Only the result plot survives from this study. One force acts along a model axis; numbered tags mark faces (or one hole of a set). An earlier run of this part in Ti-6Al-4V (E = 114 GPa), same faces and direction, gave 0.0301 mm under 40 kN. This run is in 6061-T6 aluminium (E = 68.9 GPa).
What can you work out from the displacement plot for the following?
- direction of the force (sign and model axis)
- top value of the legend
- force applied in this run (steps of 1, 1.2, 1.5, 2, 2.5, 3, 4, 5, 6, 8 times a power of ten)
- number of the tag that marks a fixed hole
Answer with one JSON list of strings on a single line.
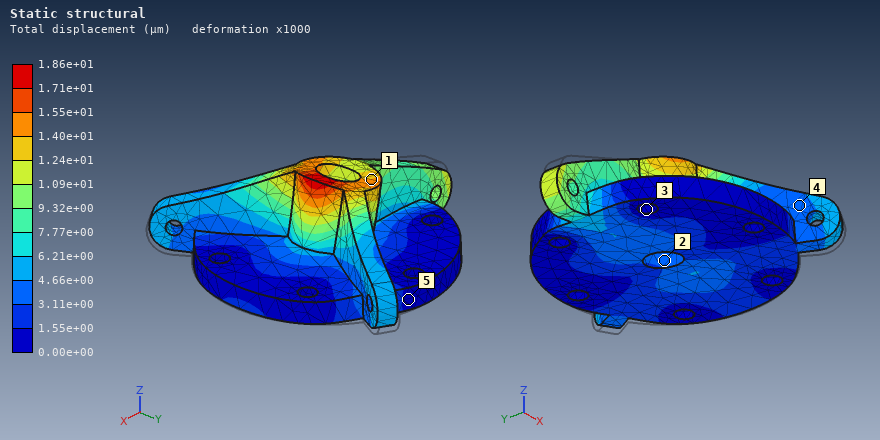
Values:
["-X", "1.86e+01 µm", "15 kN", "3"]
